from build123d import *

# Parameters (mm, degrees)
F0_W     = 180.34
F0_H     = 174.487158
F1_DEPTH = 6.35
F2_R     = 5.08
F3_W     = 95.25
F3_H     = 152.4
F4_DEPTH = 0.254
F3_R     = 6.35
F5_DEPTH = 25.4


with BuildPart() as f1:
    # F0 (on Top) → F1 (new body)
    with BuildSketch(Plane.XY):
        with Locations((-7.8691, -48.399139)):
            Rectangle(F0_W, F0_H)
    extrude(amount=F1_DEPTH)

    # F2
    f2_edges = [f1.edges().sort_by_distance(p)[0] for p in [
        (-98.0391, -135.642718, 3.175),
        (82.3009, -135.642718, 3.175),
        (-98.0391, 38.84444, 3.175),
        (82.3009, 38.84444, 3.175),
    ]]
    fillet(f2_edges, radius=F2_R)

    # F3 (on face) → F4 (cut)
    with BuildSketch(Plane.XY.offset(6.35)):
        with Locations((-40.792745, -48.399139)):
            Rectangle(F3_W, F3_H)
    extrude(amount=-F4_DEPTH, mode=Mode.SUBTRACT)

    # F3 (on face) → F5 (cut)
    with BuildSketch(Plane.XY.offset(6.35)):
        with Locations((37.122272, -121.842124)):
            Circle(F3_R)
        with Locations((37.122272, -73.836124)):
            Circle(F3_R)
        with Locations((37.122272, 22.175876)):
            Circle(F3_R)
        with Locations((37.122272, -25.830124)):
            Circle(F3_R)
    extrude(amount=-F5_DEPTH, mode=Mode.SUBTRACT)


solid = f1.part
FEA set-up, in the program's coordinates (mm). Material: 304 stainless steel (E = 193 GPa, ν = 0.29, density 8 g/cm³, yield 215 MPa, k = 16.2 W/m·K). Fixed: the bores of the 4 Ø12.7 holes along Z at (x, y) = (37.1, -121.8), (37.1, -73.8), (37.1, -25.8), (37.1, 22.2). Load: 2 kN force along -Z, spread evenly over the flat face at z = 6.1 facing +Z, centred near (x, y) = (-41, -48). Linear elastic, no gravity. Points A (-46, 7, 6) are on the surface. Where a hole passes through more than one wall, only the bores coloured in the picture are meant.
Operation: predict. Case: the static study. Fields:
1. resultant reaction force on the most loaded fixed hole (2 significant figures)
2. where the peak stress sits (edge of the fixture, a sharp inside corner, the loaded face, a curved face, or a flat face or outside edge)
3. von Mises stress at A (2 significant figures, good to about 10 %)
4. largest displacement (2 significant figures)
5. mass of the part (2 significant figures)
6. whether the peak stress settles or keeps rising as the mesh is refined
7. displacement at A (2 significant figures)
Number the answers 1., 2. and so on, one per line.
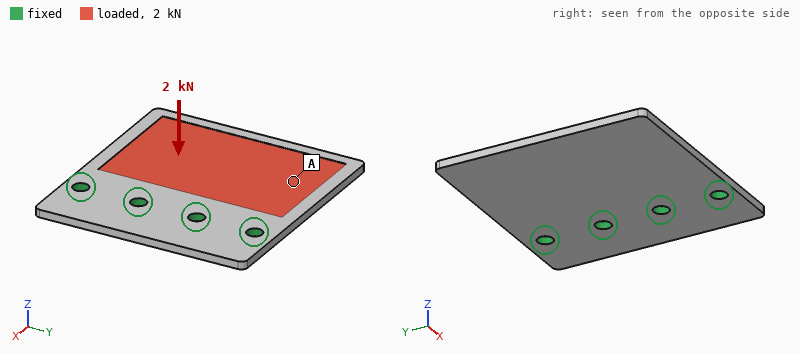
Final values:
1. 700 N
2. edge of the fixture
3. 19 MPa
4. 0.92 mm
5. 1.5 kg
6. keeps rising
7. 0.44 mm
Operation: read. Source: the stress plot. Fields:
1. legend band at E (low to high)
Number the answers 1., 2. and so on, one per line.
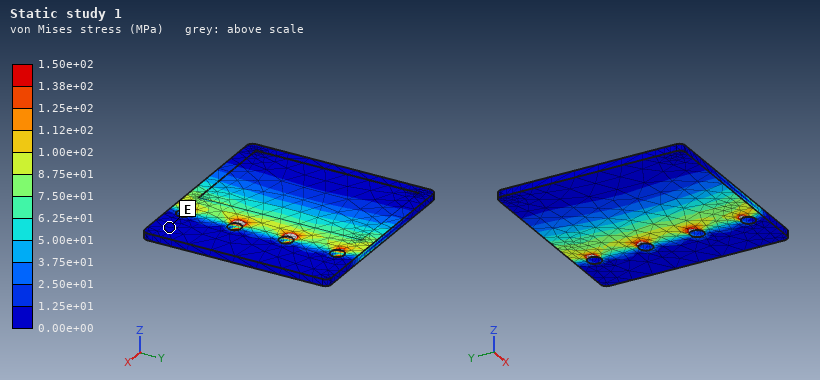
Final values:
1. 0.00e+00 to 1.25e+01 MPa
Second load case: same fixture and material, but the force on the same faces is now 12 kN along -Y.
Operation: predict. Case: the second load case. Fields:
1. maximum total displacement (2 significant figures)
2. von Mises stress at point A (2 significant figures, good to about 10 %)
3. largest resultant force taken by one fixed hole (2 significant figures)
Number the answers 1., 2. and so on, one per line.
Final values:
1. 0.13 mm
2. 19 MPa
3. 6.3 kN
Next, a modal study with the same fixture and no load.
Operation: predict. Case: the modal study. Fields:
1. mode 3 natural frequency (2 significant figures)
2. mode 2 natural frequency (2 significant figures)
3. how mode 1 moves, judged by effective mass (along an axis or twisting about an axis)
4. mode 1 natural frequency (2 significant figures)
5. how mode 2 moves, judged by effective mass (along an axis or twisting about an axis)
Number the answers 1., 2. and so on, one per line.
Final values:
1. 1400 Hz
2. 580 Hz
3. along Z
4. 290 Hz
5. twisting about X
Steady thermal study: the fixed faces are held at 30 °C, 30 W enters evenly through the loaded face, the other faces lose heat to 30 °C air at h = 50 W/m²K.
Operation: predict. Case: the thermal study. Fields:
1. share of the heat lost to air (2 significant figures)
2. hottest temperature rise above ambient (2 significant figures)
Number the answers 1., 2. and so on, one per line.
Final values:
1. 83 %
2. 25 K
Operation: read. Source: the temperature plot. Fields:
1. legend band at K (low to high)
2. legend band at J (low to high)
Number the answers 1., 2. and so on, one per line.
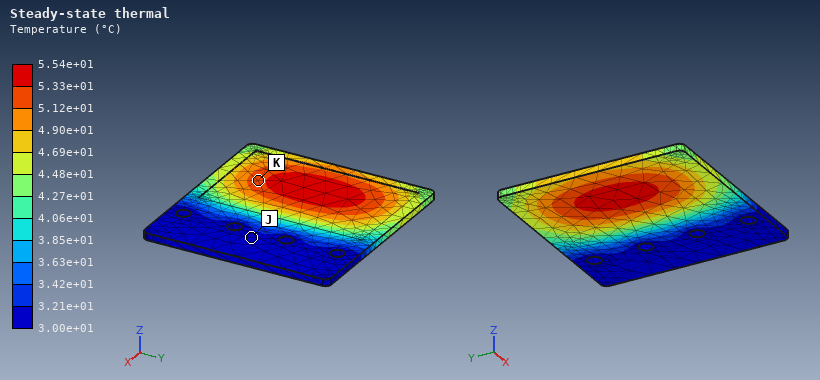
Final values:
1. 5.12e+01 to 5.33e+01 °C
2. 3.00e+01 to 3.21e+01 °C
